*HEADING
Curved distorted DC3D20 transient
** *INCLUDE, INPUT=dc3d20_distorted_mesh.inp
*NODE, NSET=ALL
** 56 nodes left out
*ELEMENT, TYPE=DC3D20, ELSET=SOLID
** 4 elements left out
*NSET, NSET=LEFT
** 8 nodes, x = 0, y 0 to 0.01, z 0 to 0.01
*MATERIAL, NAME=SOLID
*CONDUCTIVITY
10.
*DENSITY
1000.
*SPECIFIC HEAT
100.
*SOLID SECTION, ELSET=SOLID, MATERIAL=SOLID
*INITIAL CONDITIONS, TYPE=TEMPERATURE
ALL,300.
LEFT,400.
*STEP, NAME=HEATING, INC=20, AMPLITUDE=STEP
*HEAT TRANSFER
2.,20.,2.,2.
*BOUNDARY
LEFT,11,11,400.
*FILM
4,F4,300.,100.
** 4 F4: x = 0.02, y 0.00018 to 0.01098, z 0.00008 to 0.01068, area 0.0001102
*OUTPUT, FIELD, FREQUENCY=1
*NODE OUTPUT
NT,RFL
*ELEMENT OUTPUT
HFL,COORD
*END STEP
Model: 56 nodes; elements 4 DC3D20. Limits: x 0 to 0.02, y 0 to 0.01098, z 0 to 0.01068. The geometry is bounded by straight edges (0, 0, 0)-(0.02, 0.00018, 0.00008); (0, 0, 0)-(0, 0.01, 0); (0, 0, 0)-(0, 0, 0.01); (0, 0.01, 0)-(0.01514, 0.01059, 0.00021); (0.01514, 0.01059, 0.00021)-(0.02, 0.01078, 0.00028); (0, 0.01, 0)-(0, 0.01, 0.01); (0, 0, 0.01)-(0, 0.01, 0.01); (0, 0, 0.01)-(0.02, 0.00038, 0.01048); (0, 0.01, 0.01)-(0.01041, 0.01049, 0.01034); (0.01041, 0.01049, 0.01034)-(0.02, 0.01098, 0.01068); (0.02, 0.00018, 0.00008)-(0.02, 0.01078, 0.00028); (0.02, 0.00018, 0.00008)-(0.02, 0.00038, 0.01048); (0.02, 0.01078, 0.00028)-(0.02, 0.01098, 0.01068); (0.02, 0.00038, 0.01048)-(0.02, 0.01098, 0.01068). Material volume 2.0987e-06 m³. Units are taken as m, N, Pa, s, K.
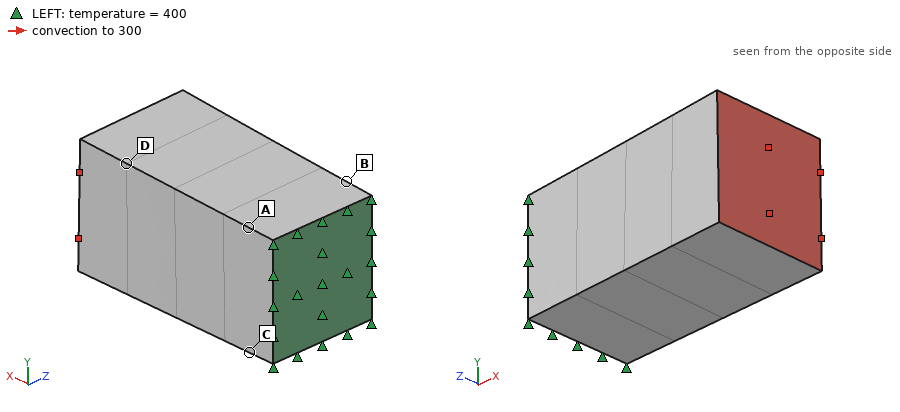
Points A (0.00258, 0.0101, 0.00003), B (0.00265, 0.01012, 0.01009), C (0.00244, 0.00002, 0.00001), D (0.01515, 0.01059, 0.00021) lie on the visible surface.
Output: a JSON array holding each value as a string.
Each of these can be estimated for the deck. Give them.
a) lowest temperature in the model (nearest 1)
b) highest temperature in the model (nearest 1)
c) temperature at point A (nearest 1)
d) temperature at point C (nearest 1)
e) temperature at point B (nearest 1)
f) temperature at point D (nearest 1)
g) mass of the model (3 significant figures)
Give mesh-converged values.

["382 K", "400 K", "398 K", "398 K", "397 K", "387 K", "0.00210 kg"]
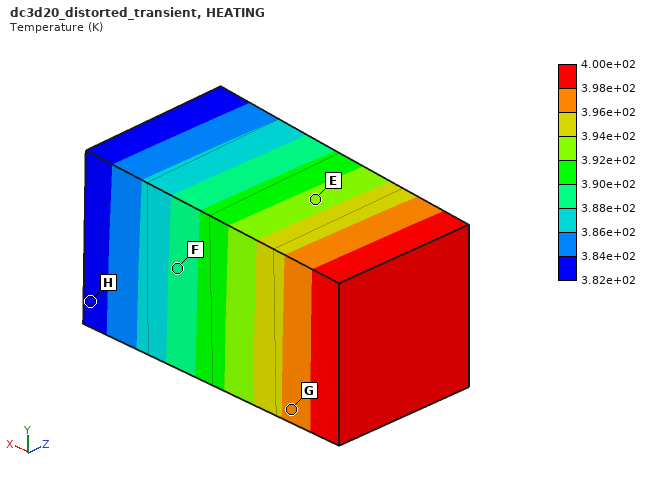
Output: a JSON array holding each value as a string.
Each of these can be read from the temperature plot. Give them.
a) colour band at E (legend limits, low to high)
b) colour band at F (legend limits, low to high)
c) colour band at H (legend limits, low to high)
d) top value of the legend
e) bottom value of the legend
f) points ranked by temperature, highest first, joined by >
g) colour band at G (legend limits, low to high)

["3.92e+02 to 3.94e+02 K", "3.88e+02 to 3.90e+02 K", "3.82e+02 to 3.84e+02 K", "4.00e+02 K", "3.82e+02 K", "G > E > F > H", "3.96e+02 to 3.98e+02 K"]
